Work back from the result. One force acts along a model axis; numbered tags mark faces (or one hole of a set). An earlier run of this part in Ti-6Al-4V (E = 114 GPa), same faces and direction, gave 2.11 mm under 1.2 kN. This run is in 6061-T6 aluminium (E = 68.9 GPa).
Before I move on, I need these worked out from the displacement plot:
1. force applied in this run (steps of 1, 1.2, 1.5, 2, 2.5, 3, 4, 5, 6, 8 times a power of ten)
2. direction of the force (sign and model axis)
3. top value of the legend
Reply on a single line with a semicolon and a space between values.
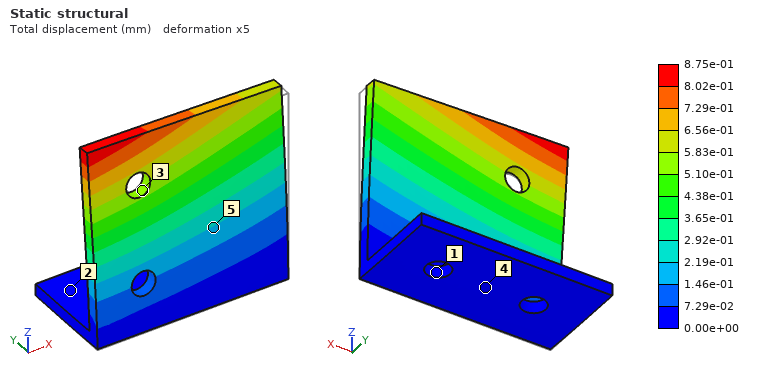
300 N; +Y; 8.75e-01 mm
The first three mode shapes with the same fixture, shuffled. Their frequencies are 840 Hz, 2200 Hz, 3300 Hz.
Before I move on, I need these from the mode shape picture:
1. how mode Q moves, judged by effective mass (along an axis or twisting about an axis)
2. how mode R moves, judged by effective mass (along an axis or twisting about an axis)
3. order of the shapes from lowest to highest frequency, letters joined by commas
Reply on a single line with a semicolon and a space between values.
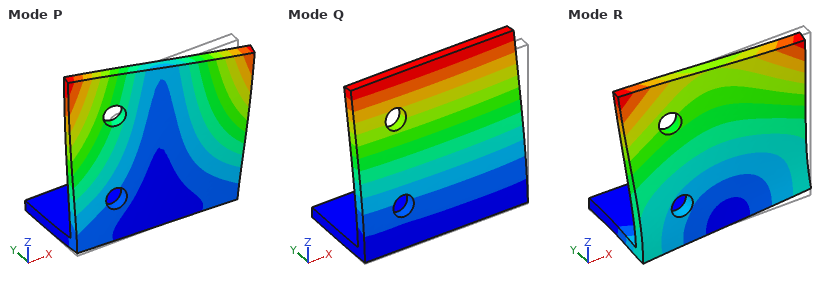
along Y; along X; Q, P, R
